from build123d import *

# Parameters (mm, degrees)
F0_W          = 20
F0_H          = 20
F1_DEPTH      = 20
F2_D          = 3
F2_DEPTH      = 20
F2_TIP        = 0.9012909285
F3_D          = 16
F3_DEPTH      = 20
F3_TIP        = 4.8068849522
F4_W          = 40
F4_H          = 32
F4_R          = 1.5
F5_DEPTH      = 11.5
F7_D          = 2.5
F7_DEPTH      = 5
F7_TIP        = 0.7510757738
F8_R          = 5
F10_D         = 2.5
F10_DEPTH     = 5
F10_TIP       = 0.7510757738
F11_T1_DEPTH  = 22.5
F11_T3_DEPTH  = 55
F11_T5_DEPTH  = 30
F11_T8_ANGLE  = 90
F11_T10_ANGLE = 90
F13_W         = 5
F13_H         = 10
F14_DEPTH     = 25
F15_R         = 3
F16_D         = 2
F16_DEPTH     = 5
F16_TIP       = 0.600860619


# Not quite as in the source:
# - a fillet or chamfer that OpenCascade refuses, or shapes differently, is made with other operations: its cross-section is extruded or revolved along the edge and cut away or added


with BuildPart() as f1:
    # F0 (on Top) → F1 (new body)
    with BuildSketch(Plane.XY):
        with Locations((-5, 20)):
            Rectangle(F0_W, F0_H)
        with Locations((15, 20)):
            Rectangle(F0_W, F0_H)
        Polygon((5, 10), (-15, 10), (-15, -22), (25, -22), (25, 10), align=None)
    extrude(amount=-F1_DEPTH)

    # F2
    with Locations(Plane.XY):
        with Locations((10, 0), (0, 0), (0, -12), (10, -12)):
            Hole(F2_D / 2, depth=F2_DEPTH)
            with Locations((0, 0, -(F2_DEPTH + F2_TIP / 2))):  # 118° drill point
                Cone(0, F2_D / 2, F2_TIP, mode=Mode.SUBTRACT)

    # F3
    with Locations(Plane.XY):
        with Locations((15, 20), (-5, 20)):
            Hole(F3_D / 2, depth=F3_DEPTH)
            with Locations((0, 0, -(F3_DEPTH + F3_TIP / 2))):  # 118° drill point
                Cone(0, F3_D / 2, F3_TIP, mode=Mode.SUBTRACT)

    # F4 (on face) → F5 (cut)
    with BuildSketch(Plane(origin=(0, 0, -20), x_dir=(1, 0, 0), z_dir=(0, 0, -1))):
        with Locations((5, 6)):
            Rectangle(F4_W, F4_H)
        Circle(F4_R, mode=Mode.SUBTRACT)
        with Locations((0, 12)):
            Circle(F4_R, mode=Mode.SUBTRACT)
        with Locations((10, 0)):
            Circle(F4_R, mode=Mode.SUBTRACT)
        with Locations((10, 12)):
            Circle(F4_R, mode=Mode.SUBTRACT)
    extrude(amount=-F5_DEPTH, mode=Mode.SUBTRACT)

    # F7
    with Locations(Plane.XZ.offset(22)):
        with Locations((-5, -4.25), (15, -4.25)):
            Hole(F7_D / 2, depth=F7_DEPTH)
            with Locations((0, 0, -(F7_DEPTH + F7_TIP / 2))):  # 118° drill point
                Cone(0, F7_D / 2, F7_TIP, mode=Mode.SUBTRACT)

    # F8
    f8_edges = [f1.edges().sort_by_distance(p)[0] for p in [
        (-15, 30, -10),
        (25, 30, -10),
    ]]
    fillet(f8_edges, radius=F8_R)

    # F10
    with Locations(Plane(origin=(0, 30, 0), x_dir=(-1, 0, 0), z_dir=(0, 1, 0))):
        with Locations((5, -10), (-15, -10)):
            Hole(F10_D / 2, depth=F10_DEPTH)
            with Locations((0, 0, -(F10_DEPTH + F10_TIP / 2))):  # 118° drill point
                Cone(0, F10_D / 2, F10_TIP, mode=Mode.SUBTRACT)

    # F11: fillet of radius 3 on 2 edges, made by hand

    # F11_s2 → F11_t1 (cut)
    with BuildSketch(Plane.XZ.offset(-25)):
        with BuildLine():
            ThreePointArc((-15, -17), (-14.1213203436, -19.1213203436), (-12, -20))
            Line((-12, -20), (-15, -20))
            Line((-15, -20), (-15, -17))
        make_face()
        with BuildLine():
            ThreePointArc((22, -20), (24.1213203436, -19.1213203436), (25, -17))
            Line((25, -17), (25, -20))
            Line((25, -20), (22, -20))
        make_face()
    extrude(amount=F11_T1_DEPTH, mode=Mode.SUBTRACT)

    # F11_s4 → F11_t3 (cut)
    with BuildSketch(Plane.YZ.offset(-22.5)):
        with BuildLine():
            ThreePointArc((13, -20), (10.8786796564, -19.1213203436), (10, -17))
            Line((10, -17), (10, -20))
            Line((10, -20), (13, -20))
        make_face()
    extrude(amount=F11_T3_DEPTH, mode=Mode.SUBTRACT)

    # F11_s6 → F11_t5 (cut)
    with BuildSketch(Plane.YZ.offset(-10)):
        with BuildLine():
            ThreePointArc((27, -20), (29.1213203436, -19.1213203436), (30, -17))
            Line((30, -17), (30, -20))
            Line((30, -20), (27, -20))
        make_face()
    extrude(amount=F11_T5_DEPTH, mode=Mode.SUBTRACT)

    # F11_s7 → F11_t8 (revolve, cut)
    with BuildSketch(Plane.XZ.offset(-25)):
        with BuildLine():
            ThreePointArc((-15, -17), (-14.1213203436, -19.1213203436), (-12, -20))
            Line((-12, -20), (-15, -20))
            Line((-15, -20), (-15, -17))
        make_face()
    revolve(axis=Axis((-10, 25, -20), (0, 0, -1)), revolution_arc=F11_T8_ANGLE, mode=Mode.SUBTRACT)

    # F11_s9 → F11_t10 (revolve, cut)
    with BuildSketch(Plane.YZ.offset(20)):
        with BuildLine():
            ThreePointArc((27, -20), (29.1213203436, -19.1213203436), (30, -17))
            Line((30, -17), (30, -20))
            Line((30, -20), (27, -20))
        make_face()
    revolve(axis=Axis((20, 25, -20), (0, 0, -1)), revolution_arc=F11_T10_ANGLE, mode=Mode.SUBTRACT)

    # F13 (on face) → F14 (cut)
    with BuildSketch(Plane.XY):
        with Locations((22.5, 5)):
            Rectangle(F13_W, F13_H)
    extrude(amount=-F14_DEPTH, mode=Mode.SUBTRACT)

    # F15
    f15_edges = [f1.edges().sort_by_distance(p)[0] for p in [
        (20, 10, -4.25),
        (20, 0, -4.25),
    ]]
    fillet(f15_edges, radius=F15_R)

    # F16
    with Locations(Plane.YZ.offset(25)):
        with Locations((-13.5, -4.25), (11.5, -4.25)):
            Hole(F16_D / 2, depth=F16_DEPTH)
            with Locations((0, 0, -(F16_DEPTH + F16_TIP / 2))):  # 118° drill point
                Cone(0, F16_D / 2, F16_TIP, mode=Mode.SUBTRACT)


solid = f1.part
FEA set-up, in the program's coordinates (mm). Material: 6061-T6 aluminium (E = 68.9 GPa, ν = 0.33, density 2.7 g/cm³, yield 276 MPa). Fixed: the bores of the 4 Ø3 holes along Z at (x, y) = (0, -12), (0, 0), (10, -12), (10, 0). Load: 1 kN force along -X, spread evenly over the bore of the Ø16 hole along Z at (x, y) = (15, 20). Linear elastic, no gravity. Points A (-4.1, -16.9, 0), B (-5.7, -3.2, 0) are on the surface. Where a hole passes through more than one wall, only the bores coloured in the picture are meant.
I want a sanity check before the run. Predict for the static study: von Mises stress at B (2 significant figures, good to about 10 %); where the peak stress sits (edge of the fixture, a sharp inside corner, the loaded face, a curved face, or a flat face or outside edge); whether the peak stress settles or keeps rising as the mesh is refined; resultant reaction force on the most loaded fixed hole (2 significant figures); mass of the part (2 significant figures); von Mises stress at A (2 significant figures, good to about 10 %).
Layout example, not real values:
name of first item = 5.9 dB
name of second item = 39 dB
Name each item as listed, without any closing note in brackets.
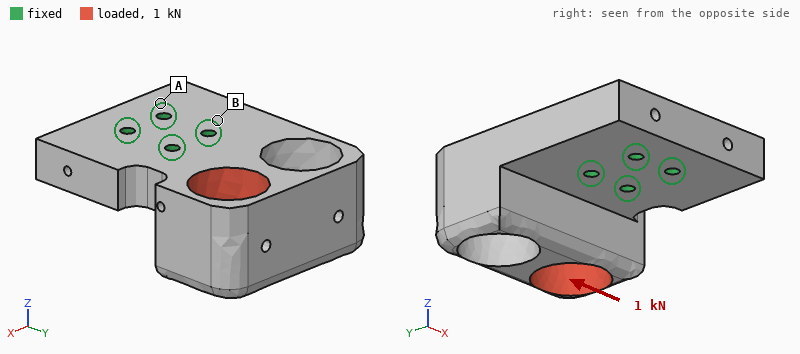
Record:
von Mises stress at B = 11 MPa
where the peak stress sits = edge of the fixture
whether the peak stress settles or keeps rising as the mesh is refined = keeps rising
resultant reaction force on the most loaded fixed hole = 1.1 kN
mass of the part = 48 g
von Mises stress at A = 4.1 MPa
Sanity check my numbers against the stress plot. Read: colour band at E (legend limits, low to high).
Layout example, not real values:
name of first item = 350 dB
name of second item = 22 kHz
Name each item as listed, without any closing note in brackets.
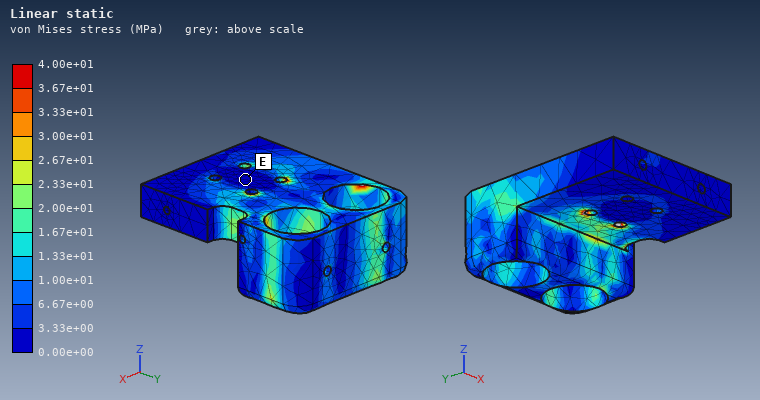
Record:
colour band at E = 0.00e+00 to 3.33e+00 MPa
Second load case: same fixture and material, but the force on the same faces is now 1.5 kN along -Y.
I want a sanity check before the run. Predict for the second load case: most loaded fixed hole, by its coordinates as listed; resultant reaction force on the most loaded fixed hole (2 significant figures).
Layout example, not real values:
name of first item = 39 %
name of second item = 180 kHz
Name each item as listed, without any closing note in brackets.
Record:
most loaded fixed hole, by its coordinates as listed = (10, 0)
resultant reaction force on the most loaded fixed hole = 1.2 kN
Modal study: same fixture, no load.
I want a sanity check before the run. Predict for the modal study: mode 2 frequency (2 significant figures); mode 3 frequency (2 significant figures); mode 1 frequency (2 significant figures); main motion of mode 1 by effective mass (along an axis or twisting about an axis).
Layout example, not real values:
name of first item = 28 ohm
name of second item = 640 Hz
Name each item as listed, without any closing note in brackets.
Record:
mode 2 frequency = 8100 Hz
mode 3 frequency = 8400 Hz
mode 1 frequency = 5100 Hz
main motion of mode 1 by effective mass = along Z
